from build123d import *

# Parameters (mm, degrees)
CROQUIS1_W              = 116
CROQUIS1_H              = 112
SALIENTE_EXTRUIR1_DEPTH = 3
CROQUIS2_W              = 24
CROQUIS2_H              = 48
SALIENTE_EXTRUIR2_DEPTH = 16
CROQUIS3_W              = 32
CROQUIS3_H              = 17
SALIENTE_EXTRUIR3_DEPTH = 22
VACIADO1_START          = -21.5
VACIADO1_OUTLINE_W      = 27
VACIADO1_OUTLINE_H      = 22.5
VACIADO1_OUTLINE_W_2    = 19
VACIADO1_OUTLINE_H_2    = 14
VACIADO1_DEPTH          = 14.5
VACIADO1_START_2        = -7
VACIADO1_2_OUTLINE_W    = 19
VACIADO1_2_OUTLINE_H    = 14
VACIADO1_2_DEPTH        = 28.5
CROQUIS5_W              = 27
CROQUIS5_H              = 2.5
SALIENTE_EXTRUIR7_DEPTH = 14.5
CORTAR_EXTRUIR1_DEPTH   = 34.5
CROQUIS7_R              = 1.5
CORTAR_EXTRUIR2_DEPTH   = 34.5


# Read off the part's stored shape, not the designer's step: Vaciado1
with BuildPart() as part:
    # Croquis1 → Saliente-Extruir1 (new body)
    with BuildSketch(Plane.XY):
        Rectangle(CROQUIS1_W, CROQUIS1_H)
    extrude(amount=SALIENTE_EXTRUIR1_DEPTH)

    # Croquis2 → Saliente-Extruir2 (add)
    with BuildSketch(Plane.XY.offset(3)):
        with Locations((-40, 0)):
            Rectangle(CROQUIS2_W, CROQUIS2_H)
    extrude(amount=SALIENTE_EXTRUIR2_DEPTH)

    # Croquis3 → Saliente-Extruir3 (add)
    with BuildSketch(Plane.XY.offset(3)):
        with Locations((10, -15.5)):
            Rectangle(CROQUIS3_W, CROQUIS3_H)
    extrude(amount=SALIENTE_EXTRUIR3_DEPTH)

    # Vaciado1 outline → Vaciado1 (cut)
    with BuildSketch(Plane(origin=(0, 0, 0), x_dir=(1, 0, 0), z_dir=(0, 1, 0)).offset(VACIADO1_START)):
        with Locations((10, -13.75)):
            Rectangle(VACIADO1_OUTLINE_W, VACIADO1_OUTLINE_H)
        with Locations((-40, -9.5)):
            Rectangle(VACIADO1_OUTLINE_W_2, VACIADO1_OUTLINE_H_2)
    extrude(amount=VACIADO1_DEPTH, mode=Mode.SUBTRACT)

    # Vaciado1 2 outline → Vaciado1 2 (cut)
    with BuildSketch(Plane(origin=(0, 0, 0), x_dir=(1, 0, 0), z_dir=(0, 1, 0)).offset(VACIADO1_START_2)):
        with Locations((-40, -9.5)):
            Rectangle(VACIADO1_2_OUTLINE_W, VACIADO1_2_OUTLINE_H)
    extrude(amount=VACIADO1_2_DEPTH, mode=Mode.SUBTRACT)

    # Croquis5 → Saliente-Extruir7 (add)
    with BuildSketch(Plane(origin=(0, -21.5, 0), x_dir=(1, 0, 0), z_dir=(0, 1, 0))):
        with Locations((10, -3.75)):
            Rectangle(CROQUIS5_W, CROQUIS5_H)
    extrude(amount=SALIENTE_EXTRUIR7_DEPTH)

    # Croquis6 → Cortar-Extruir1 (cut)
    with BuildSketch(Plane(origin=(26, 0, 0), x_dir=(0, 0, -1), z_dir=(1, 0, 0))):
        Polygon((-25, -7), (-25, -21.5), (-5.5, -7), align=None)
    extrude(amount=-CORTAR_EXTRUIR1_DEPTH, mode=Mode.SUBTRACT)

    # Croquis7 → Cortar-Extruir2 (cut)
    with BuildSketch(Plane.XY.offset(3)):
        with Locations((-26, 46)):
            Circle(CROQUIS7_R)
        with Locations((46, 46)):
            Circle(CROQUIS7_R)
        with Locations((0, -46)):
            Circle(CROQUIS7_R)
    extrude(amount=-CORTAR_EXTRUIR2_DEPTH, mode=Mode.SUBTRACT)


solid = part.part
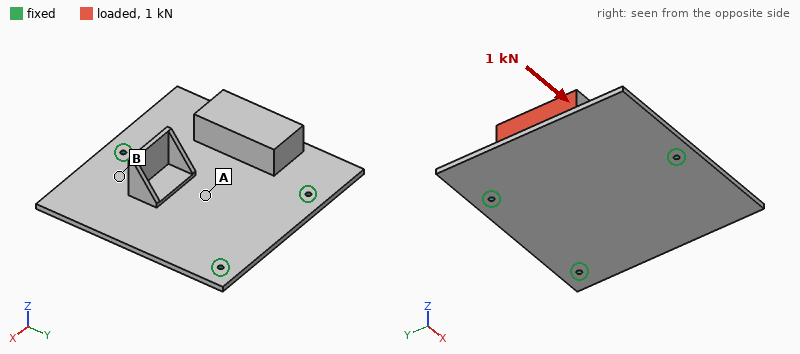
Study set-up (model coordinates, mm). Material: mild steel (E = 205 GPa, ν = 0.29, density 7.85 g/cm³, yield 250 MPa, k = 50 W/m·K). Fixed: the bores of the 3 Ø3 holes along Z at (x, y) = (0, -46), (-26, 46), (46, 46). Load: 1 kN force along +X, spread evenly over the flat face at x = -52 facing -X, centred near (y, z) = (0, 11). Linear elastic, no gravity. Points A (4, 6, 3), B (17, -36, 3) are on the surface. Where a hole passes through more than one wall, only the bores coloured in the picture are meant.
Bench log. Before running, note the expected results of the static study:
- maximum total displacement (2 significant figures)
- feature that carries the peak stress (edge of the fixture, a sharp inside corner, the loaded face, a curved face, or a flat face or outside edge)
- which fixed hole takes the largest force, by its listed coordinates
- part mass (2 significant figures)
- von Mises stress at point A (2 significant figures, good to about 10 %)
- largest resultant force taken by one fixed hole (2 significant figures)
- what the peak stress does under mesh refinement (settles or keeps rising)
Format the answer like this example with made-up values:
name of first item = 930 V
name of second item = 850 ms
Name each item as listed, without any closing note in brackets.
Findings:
maximum total displacement = 0.17 mm
feature that carries the peak stress = edge of the fixture
which fixed hole takes the largest force, by its listed coordinates = (0, -46)
part mass = 390 g
von Mises stress at point A = 15 MPa
largest resultant force taken by one fixed hole = 460 N
what the peak stress does under mesh refinement = keeps rising
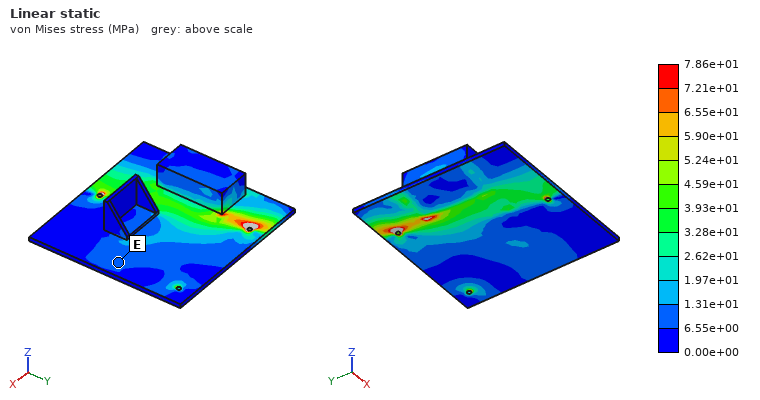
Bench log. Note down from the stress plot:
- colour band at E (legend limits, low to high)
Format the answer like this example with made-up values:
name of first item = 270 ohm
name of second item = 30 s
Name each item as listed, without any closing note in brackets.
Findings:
colour band at E = 6.55e+00 to 1.31e+01 MPa
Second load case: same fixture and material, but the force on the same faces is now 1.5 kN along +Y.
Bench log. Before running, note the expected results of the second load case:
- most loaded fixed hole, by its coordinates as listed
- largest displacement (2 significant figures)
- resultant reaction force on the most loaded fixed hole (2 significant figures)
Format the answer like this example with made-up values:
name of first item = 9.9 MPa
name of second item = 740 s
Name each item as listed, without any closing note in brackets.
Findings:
most loaded fixed hole, by its coordinates as listed = (-26, 46)
largest displacement = 0.12 mm
resultant reaction force on the most loaded fixed hole = 1.0 kN
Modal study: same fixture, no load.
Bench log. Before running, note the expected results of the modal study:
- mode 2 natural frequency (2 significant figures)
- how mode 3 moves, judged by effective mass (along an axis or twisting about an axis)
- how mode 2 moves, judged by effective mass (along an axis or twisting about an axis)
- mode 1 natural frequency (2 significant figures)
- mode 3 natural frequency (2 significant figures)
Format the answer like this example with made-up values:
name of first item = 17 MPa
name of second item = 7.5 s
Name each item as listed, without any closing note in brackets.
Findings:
mode 2 natural frequency = 970 Hz
how mode 3 moves, judged by effective mass = along Z
how mode 2 moves, judged by effective mass = along Z
mode 1 natural frequency = 690 Hz
mode 3 natural frequency = 1600 Hz
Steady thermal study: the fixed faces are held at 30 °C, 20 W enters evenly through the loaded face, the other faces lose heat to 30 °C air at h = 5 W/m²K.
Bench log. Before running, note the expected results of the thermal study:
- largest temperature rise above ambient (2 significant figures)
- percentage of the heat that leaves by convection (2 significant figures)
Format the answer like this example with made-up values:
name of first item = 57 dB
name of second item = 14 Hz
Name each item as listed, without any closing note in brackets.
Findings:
largest temperature rise above ambient = 73 K
percentage of the heat that leaves by convection = 24 %
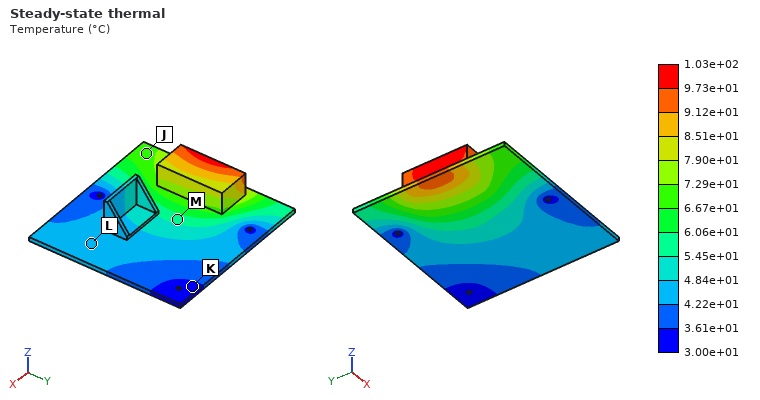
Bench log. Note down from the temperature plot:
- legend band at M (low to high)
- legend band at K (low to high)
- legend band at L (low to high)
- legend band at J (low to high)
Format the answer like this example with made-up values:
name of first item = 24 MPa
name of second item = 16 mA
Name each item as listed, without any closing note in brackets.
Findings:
legend band at M = 5.45e+01 to 6.06e+01 °C
legend band at K = 3.00e+01 to 3.61e+01 °C
legend band at L = 4.22e+01 to 4.84e+01 °C
legend band at J = 6.67e+01 to 7.29e+01 °C
